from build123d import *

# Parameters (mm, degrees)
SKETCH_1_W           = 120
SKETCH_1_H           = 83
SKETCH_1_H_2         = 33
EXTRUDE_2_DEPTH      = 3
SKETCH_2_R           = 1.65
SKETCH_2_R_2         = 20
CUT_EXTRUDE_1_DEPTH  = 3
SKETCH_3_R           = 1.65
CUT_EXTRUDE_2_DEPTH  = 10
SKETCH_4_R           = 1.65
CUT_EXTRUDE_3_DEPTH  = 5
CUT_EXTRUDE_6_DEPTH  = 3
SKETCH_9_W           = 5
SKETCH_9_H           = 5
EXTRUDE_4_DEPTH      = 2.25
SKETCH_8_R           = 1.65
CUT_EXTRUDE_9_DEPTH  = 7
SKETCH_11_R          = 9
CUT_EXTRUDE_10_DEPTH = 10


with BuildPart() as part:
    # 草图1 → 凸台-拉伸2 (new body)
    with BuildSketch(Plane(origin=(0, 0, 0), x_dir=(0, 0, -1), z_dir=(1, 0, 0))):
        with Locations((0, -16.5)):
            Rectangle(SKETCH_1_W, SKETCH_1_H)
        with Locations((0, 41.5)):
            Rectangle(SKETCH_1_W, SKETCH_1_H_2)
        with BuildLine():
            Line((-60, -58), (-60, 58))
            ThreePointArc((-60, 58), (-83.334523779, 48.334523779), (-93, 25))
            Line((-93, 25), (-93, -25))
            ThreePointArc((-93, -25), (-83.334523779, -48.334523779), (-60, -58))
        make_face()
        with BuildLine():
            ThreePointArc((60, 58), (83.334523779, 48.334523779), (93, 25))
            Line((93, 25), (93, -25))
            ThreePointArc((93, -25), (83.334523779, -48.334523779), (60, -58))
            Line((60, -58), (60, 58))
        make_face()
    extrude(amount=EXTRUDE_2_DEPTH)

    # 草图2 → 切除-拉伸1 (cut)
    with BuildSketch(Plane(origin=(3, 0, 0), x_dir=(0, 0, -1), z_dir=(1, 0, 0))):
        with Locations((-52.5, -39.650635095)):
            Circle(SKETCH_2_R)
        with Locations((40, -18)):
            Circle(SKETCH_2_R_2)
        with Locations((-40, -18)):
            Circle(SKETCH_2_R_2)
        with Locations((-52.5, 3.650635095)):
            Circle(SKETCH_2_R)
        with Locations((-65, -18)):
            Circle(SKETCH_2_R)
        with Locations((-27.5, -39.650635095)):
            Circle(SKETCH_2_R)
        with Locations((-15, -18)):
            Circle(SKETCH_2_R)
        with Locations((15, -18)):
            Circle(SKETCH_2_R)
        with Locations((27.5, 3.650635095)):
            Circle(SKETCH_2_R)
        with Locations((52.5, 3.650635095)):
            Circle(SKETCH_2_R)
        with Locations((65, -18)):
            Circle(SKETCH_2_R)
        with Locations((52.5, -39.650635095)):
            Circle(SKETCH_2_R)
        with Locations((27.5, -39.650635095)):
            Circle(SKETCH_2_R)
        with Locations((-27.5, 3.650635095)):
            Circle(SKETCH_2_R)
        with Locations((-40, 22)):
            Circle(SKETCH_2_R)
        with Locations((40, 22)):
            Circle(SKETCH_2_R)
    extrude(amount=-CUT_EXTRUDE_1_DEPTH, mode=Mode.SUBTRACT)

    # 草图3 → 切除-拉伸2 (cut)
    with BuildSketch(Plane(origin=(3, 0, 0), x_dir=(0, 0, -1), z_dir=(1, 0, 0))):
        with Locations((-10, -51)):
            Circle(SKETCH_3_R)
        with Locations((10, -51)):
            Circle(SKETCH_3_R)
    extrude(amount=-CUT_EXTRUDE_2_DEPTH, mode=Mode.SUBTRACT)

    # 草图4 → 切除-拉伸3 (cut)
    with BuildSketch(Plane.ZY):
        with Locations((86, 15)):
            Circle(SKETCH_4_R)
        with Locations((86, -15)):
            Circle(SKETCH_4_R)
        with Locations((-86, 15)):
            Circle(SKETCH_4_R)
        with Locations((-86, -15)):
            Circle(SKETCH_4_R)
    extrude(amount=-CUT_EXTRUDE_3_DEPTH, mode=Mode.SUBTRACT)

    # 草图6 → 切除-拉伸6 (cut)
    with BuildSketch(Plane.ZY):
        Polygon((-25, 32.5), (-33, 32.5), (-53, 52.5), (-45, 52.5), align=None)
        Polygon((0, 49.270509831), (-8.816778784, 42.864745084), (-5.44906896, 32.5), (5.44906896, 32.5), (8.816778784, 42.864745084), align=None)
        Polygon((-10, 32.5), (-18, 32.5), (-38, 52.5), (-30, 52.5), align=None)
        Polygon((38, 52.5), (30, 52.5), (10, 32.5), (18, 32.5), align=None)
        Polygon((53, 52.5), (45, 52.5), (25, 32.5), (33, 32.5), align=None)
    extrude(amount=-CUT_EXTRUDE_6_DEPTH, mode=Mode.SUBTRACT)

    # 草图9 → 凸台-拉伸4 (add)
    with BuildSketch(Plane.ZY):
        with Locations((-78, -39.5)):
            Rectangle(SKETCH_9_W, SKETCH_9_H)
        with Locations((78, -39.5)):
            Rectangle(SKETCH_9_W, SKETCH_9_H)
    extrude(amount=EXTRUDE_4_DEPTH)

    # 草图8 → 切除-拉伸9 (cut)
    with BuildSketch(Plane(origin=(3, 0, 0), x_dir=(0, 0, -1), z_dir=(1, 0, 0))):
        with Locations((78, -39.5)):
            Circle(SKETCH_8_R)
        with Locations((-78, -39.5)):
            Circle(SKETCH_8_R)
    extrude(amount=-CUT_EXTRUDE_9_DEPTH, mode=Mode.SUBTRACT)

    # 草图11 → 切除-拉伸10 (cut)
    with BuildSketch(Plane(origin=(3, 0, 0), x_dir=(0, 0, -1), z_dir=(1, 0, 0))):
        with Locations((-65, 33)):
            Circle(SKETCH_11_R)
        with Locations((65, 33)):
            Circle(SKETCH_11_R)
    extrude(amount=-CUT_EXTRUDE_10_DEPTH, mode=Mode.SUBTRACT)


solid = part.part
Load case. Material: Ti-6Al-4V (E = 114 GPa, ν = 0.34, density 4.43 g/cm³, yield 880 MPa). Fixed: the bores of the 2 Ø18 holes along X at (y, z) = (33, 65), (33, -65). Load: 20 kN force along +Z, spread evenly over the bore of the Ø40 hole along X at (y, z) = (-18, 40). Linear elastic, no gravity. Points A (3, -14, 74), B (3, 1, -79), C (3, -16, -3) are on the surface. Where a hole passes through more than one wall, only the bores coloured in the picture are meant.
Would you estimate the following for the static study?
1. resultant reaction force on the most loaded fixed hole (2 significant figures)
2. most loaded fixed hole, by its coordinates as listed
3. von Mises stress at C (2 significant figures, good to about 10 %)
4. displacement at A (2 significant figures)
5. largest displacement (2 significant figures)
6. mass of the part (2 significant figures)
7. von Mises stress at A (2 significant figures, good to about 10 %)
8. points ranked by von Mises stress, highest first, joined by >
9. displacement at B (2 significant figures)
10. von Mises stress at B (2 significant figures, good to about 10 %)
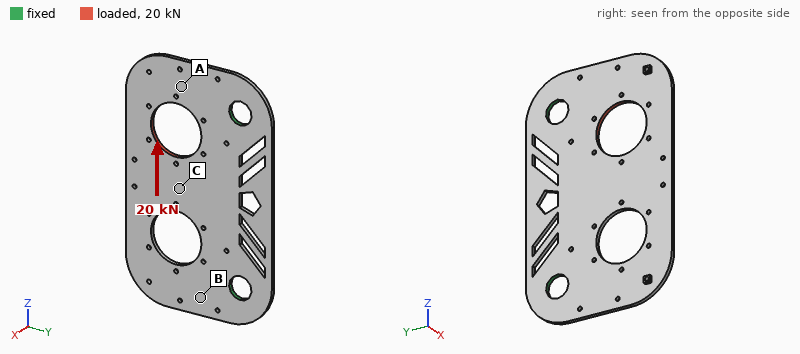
13 kN
(33, 65)
110 MPa
0.11 mm
0.16 mm
220 g
74 MPa
C > A > B
0.036 mm
36 MPa
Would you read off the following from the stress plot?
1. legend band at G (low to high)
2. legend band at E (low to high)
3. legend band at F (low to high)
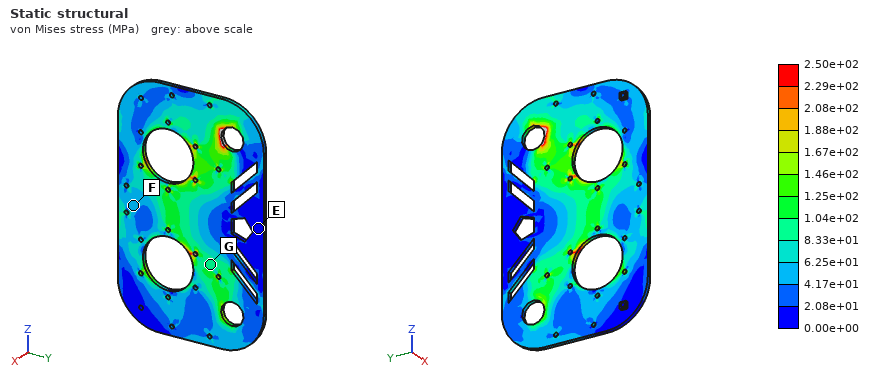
8.33e+01 to 1.04e+02 MPa
0.00e+00 to 2.08e+01 MPa
4.17e+01 to 6.25e+01 MPa
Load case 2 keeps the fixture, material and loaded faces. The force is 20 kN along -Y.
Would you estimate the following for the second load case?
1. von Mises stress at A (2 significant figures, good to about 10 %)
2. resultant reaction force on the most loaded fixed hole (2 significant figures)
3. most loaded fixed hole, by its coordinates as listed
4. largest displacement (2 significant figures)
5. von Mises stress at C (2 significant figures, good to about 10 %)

97 MPa
16 kN
(33, 65)
0.11 mm
44 MPa
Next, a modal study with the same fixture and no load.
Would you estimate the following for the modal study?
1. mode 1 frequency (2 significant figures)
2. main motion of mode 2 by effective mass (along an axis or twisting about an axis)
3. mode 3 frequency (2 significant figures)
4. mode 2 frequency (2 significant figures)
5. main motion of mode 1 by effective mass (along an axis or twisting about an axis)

300 Hz
twisting about Y
810 Hz
520 Hz
along X
